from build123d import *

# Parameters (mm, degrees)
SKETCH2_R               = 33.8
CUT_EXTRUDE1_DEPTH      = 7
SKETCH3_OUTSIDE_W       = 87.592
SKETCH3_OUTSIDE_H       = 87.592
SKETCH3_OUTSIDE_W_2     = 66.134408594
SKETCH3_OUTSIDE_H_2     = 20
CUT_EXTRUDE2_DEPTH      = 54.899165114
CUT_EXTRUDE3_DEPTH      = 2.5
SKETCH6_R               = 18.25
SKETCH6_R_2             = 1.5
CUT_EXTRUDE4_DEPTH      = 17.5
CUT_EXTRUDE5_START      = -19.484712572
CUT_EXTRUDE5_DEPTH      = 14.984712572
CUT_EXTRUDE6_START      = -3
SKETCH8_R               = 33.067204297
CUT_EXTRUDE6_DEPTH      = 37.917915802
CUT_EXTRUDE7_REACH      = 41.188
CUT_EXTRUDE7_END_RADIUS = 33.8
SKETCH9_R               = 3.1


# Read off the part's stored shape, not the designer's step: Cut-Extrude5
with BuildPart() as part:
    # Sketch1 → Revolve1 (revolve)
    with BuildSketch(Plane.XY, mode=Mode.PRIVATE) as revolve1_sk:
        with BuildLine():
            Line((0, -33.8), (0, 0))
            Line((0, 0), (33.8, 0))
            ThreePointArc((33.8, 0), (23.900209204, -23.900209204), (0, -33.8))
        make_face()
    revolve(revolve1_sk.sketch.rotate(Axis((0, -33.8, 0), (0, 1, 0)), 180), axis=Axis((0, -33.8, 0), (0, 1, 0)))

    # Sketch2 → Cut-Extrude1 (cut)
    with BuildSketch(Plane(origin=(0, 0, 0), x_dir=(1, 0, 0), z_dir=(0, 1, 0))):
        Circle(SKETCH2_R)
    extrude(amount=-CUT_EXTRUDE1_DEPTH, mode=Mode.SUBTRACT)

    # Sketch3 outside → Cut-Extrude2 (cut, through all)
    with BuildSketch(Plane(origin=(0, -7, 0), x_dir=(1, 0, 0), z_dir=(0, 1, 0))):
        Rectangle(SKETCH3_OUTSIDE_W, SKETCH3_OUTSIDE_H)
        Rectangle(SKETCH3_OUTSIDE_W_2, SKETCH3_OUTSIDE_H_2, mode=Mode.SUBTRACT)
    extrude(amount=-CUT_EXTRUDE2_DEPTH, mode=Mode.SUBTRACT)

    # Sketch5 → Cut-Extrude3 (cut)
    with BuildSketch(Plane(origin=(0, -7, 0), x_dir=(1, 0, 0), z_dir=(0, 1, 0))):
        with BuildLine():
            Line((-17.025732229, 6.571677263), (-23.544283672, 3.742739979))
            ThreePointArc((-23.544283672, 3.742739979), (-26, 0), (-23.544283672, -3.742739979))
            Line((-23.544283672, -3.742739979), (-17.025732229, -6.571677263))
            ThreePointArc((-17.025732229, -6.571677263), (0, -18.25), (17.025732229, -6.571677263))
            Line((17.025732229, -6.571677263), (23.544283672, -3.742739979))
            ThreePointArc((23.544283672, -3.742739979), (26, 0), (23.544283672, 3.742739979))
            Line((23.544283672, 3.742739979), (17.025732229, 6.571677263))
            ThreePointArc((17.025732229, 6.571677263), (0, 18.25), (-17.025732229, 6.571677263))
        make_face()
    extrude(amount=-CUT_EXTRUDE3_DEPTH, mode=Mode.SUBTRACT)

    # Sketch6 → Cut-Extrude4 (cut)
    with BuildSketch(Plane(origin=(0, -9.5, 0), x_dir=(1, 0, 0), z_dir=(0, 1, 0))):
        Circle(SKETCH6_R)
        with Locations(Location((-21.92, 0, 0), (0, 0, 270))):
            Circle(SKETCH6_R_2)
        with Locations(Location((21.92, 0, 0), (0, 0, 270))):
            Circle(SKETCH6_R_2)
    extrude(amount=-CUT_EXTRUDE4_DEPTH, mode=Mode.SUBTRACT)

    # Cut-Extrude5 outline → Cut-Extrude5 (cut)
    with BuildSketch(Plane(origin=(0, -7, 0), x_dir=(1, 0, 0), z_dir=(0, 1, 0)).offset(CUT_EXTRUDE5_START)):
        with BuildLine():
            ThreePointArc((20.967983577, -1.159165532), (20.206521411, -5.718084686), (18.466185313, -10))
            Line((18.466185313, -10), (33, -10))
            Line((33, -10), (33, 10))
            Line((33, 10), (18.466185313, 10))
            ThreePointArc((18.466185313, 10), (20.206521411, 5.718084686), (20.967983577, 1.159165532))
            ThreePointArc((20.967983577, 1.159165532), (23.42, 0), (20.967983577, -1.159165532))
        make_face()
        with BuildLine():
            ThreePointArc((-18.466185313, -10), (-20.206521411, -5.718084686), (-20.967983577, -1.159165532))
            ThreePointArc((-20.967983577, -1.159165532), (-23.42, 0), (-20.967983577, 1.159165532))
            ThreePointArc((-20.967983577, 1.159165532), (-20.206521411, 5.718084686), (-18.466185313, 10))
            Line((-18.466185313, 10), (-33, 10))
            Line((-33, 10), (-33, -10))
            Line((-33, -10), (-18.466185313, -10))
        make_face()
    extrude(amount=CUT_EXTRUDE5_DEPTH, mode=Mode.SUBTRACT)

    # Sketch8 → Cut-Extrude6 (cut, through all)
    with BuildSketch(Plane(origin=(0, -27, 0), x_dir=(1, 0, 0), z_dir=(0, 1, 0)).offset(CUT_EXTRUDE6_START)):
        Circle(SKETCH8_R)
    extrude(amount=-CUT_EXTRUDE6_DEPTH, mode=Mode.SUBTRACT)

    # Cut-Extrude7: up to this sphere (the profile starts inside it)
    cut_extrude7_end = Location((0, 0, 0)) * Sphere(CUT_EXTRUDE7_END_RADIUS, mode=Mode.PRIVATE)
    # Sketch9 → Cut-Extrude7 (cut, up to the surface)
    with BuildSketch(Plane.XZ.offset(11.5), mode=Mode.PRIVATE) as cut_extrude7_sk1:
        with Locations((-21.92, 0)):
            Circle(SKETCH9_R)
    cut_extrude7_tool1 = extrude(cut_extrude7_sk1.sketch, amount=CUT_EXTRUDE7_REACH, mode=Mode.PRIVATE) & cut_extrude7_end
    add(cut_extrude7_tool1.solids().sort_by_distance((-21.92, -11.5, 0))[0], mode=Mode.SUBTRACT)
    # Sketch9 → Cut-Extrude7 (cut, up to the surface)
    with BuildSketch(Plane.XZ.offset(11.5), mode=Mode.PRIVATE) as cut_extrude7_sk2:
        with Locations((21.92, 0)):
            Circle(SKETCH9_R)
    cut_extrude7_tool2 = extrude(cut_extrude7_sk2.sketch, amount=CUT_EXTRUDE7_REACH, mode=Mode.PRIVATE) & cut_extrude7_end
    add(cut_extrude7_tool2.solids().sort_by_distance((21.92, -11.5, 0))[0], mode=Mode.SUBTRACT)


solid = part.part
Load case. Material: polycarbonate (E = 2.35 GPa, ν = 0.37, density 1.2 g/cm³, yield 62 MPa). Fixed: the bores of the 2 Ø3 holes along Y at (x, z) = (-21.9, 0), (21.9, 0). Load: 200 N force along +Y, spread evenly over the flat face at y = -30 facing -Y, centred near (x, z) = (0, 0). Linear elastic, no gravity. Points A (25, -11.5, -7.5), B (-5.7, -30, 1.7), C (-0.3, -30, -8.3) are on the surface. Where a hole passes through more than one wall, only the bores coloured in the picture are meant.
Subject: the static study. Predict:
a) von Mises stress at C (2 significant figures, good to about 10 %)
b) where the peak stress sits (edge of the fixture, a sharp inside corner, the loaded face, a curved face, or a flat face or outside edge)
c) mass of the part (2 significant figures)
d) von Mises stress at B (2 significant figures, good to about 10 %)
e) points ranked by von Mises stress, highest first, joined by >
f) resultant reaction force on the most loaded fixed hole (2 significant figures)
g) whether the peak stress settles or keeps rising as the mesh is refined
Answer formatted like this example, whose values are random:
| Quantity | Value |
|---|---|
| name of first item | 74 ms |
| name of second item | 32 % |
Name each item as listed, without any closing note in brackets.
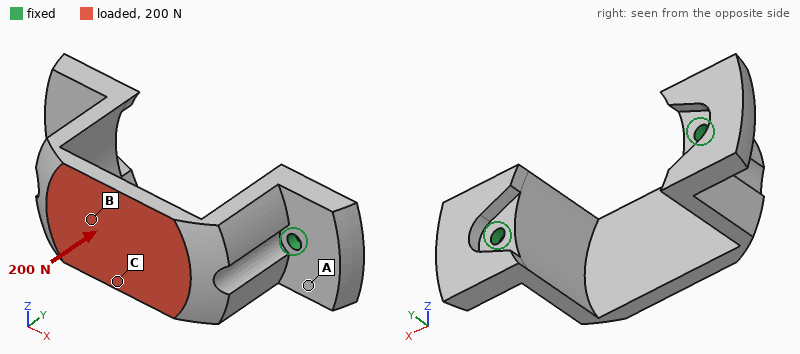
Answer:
| Quantity | Value |
|---|---|
| von Mises stress at C | 23 MPa |
| where the peak stress sits | a sharp inside corner |
| mass of the part | 7.0 g |
| von Mises stress at B | 17 MPa |
| points ranked by von Mises stress, highest first, joined by > | C > B > A |
| resultant reaction force on the most loaded fixed hole | 110 N |
| whether the peak stress settles or keeps rising as the mesh is refined | keeps rising |
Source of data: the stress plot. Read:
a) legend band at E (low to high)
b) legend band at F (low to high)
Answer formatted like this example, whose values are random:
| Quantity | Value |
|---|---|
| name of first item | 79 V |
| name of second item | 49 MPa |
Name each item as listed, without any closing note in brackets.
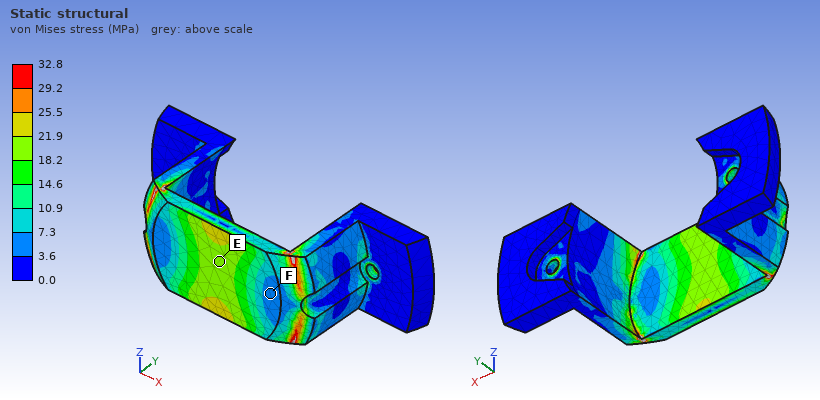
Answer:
| Quantity | Value |
|---|---|
| legend band at E | 18.2 to 21.9 MPa |
| legend band at F | 3.6 to 7.3 MPa |
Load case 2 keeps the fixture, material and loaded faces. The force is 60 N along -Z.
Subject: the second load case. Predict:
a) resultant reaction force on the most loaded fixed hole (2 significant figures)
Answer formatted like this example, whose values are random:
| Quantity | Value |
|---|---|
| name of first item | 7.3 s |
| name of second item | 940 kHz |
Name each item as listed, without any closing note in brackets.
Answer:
| Quantity | Value |
|---|---|
| resultant reaction force on the most loaded fixed hole | 30 N |
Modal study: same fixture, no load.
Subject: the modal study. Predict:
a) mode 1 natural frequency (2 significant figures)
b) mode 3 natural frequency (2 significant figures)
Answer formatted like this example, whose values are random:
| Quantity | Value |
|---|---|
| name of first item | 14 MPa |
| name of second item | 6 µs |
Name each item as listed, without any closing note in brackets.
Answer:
| Quantity | Value |
|---|---|
| mode 1 natural frequency | 930 Hz |
| mode 3 natural frequency | 1700 Hz |
